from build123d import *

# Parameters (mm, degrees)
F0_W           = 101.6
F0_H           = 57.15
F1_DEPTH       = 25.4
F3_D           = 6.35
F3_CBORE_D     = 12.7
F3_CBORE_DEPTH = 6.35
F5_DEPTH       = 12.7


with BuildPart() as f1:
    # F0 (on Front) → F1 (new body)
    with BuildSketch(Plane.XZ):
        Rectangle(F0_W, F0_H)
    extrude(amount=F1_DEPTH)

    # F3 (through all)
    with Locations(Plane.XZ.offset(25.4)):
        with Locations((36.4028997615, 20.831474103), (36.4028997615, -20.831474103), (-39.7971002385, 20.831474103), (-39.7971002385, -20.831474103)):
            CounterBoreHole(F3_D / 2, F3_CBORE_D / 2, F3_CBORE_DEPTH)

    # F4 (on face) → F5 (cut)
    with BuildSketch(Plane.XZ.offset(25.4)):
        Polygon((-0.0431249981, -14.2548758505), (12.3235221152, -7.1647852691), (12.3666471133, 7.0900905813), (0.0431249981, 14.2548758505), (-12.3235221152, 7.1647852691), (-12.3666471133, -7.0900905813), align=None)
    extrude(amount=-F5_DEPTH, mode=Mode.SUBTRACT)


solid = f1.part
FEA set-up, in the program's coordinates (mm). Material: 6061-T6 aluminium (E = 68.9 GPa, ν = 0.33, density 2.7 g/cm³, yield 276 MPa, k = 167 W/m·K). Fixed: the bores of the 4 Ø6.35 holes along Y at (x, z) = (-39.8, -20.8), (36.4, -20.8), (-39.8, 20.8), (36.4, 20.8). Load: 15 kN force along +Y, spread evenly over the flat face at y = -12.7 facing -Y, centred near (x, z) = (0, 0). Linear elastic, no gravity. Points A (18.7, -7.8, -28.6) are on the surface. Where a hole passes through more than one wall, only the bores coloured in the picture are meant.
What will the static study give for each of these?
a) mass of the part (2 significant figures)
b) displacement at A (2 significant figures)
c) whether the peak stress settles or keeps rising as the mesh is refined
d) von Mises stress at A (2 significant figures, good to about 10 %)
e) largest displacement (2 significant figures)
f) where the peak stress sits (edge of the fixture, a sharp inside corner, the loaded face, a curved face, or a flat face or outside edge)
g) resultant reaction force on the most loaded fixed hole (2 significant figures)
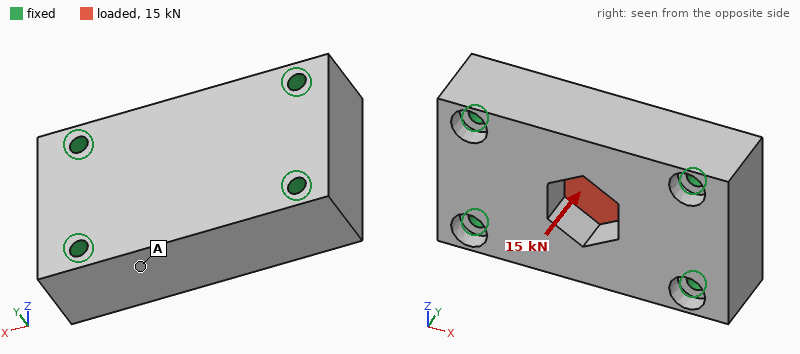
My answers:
360 g
9.9 µm
keeps rising
14 MPa
31 µm
edge of the fixture
4.0 kN
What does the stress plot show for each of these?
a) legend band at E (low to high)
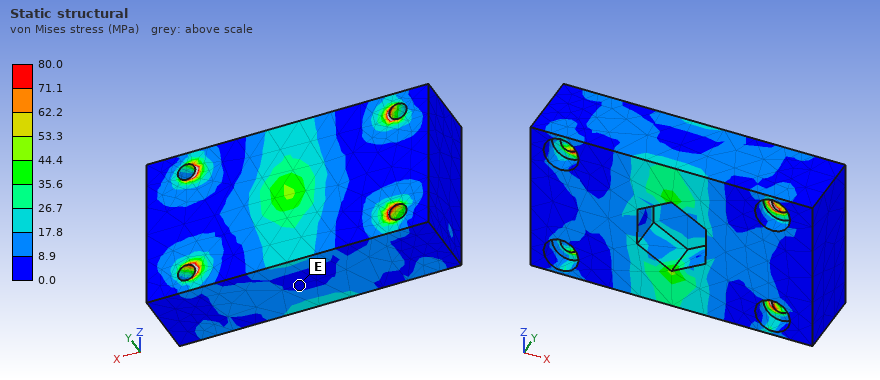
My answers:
0.0 to 8.9 MPa
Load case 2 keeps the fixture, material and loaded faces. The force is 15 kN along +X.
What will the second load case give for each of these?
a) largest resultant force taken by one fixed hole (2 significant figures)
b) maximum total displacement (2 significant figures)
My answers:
4.0 kN
12 µm
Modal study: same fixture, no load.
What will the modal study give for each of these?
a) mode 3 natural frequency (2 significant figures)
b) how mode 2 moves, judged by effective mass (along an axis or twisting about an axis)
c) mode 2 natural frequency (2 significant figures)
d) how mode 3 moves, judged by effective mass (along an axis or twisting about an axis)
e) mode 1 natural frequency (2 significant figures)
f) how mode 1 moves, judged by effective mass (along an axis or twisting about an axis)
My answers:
17 kHz
twisting about X
16 kHz
along Z
12 kHz
along Y
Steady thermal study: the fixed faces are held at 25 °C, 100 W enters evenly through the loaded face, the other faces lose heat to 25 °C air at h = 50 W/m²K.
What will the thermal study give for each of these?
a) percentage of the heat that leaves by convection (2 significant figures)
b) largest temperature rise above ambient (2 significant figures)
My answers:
3.4 %
17 K
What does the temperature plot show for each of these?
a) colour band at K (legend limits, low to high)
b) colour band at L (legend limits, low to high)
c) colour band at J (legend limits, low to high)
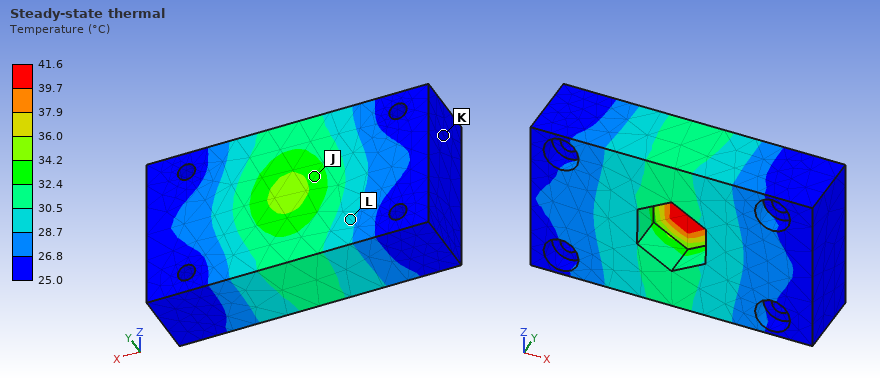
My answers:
25.0 to 26.8 °C
28.7 to 30.5 °C
32.4 to 34.2 °C
